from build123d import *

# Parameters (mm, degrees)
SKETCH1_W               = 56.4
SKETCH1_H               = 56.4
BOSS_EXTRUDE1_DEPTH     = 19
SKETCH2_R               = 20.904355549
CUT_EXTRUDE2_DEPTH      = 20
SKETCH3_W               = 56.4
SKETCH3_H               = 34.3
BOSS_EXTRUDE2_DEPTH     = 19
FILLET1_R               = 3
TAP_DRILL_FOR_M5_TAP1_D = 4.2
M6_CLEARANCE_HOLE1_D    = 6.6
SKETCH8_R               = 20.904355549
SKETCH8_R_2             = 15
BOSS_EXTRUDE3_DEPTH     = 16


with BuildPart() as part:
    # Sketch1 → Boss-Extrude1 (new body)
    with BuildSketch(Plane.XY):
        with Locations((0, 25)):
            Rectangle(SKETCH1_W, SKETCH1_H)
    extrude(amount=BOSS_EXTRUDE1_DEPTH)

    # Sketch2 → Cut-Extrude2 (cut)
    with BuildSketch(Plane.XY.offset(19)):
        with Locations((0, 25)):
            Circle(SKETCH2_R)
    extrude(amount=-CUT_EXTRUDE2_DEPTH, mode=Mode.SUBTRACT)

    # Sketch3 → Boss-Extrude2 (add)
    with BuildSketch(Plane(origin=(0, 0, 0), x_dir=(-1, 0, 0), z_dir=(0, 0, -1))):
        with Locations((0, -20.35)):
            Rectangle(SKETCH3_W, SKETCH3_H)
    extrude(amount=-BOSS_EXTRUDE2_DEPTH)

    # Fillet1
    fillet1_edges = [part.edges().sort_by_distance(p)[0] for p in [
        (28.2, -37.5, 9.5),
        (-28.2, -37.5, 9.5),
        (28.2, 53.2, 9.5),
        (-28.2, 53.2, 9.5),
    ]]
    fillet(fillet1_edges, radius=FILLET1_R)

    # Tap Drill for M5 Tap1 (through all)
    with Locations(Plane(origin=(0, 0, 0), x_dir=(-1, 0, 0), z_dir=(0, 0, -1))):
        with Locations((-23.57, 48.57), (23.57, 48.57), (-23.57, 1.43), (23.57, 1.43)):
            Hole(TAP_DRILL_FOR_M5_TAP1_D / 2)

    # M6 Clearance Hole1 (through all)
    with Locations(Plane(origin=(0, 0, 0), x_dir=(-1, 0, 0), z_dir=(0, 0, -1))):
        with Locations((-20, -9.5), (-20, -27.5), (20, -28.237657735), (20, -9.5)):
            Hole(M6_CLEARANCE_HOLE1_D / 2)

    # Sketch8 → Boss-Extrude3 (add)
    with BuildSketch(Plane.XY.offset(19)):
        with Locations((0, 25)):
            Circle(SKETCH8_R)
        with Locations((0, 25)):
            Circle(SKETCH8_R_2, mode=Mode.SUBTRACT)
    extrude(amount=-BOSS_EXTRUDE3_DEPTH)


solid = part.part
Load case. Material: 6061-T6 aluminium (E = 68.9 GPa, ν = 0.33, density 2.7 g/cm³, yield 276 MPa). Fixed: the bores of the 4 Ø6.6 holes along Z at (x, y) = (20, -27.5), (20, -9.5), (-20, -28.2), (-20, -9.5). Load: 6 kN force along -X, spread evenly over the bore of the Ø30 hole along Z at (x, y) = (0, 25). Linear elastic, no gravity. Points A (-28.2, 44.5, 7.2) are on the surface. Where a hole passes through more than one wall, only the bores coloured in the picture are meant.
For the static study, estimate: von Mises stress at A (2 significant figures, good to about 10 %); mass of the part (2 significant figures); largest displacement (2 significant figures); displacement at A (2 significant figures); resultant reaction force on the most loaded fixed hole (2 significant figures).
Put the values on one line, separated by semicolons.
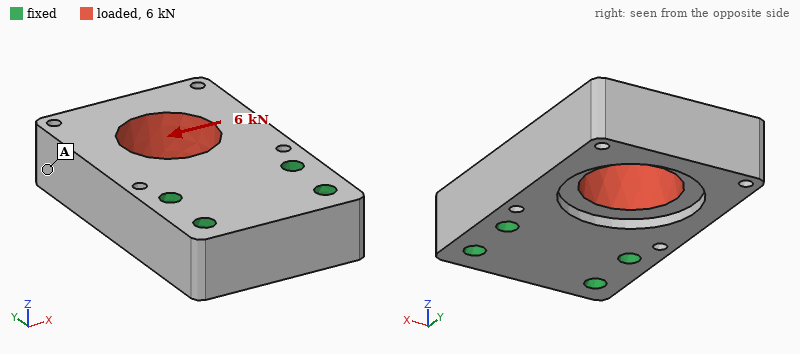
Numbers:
6.7 MPa; 210 g; 46 µm; 42 µm; 5.1 kN
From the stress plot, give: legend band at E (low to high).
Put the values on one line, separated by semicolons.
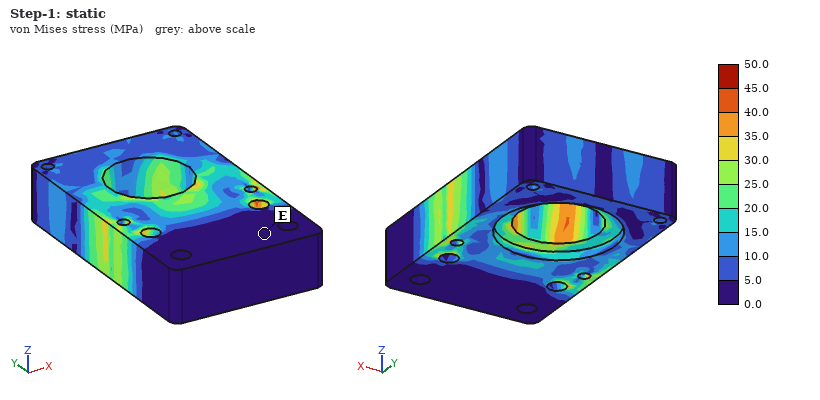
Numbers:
0.0 to 5.0 MPa
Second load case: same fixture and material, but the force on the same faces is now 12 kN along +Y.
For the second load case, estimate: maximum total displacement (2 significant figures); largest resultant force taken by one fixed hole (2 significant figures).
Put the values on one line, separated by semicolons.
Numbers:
26 µm; 5.1 kN
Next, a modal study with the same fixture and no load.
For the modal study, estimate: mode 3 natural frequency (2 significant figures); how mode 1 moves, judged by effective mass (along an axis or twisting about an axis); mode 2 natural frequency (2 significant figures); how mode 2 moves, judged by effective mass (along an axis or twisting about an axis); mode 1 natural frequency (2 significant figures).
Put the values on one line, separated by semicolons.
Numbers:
6600 Hz; along Z; 5800 Hz; along X; 3300 Hz
